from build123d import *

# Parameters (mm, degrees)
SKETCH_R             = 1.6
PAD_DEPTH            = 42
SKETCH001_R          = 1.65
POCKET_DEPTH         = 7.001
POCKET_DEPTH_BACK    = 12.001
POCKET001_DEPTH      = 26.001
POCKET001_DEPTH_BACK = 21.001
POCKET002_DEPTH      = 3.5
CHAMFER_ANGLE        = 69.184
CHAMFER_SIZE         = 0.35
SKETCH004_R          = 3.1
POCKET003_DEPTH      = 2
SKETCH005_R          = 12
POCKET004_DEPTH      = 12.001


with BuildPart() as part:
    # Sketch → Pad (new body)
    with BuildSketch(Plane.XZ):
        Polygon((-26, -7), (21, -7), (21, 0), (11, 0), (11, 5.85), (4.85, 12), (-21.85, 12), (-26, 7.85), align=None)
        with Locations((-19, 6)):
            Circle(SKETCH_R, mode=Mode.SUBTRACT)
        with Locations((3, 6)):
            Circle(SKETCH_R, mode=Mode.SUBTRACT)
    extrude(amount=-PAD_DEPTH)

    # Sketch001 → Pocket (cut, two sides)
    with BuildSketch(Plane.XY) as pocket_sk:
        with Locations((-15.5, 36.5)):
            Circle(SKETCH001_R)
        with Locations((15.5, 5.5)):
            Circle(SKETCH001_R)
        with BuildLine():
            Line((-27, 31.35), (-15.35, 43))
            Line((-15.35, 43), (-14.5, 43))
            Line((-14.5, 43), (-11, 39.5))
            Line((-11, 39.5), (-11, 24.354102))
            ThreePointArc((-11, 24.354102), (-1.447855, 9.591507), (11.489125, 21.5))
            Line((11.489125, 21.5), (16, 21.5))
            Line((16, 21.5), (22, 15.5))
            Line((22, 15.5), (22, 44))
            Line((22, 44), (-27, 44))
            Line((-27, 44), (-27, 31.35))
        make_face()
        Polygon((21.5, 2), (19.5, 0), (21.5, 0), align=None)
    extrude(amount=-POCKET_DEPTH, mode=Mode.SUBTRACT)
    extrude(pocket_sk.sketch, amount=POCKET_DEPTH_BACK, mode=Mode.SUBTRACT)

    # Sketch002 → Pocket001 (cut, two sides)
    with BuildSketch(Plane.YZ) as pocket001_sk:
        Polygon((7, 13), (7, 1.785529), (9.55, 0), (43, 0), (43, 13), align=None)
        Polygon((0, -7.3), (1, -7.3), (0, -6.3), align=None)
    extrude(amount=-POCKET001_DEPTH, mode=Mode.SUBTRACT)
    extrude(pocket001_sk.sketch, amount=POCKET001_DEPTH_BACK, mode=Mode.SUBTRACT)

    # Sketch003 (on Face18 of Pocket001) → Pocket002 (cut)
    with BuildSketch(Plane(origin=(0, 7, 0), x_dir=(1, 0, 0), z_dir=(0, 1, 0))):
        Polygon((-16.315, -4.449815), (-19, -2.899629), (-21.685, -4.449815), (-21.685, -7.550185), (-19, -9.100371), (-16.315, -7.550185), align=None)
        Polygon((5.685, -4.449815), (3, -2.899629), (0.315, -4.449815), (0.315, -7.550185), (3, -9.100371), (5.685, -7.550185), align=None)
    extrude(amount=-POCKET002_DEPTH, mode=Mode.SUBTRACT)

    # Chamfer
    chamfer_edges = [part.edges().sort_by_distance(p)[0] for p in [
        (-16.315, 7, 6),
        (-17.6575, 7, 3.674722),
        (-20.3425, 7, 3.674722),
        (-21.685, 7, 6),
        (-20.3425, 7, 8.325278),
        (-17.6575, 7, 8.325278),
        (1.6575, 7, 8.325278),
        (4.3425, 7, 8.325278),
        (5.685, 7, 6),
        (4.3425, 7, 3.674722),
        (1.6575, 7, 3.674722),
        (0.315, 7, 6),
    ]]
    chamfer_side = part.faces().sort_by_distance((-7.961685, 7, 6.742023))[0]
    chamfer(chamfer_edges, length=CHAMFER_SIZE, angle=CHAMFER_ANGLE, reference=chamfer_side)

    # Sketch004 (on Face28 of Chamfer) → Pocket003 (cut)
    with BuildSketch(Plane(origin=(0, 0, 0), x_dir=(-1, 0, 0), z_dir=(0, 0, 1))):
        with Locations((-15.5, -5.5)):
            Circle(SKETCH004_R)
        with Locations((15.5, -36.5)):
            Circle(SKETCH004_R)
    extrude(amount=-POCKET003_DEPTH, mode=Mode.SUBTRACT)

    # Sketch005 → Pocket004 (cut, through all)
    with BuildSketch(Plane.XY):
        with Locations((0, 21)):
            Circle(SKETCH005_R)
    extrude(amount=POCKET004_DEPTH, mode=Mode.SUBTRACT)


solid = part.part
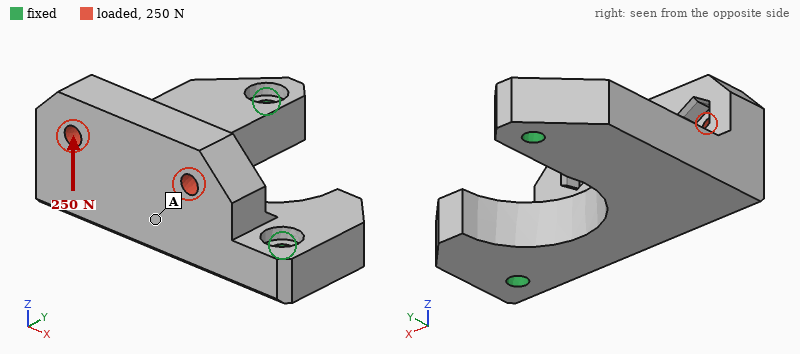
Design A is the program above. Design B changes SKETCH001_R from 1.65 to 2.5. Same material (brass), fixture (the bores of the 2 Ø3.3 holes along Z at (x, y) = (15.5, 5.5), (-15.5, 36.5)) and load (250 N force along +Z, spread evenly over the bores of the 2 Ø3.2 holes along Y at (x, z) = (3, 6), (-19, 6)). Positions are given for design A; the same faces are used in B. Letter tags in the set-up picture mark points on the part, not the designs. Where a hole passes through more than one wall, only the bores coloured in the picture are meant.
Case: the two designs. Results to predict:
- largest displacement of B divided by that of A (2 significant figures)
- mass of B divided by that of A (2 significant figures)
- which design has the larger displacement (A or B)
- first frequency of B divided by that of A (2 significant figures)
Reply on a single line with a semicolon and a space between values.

0.79; 0.99; A; 1.1
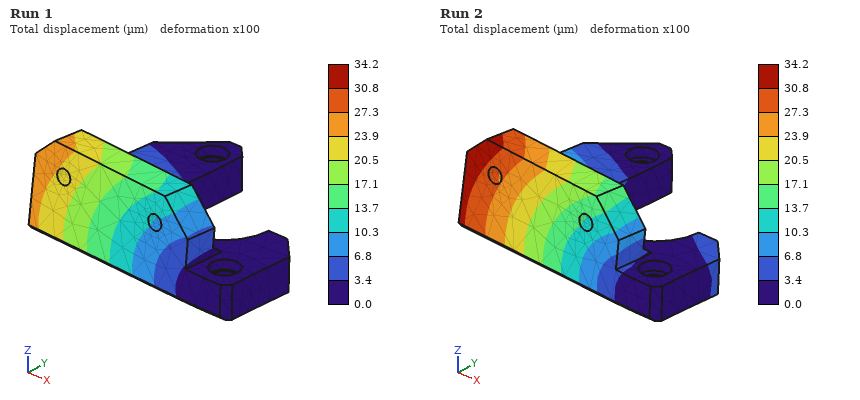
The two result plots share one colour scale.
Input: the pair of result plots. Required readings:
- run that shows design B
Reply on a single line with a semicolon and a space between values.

Run 1
